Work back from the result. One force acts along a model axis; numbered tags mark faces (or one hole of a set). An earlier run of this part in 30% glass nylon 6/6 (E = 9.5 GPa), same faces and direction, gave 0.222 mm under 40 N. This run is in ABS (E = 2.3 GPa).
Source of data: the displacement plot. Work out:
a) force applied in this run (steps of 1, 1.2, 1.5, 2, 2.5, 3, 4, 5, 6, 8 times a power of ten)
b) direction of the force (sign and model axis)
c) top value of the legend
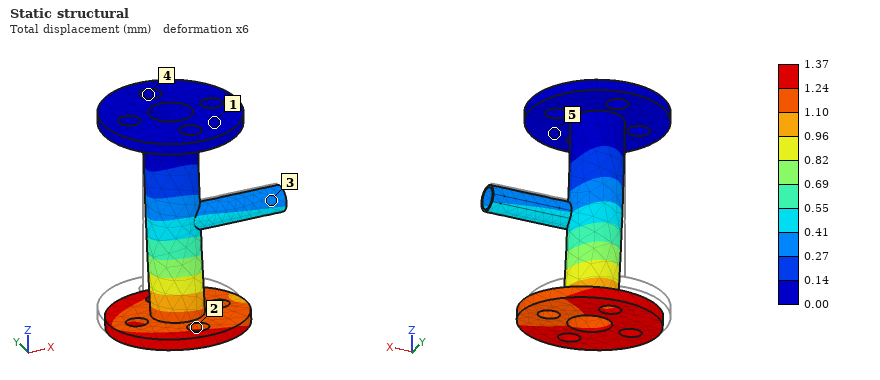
60 N
-Y
1.37 mm
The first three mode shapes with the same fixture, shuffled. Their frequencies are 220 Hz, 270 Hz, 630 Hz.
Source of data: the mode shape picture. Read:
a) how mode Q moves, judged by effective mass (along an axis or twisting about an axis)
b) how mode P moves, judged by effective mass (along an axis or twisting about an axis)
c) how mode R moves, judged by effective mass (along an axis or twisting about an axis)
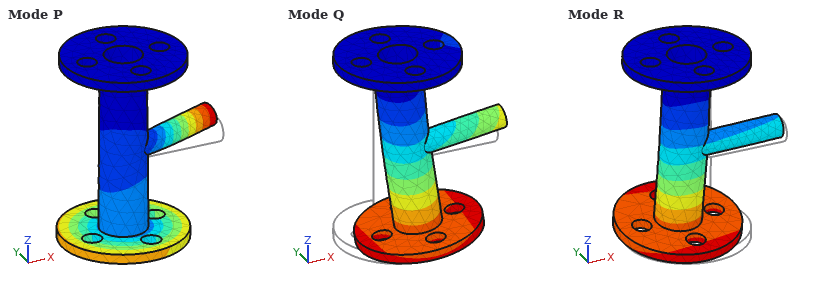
along X
twisting about Z
along Y
